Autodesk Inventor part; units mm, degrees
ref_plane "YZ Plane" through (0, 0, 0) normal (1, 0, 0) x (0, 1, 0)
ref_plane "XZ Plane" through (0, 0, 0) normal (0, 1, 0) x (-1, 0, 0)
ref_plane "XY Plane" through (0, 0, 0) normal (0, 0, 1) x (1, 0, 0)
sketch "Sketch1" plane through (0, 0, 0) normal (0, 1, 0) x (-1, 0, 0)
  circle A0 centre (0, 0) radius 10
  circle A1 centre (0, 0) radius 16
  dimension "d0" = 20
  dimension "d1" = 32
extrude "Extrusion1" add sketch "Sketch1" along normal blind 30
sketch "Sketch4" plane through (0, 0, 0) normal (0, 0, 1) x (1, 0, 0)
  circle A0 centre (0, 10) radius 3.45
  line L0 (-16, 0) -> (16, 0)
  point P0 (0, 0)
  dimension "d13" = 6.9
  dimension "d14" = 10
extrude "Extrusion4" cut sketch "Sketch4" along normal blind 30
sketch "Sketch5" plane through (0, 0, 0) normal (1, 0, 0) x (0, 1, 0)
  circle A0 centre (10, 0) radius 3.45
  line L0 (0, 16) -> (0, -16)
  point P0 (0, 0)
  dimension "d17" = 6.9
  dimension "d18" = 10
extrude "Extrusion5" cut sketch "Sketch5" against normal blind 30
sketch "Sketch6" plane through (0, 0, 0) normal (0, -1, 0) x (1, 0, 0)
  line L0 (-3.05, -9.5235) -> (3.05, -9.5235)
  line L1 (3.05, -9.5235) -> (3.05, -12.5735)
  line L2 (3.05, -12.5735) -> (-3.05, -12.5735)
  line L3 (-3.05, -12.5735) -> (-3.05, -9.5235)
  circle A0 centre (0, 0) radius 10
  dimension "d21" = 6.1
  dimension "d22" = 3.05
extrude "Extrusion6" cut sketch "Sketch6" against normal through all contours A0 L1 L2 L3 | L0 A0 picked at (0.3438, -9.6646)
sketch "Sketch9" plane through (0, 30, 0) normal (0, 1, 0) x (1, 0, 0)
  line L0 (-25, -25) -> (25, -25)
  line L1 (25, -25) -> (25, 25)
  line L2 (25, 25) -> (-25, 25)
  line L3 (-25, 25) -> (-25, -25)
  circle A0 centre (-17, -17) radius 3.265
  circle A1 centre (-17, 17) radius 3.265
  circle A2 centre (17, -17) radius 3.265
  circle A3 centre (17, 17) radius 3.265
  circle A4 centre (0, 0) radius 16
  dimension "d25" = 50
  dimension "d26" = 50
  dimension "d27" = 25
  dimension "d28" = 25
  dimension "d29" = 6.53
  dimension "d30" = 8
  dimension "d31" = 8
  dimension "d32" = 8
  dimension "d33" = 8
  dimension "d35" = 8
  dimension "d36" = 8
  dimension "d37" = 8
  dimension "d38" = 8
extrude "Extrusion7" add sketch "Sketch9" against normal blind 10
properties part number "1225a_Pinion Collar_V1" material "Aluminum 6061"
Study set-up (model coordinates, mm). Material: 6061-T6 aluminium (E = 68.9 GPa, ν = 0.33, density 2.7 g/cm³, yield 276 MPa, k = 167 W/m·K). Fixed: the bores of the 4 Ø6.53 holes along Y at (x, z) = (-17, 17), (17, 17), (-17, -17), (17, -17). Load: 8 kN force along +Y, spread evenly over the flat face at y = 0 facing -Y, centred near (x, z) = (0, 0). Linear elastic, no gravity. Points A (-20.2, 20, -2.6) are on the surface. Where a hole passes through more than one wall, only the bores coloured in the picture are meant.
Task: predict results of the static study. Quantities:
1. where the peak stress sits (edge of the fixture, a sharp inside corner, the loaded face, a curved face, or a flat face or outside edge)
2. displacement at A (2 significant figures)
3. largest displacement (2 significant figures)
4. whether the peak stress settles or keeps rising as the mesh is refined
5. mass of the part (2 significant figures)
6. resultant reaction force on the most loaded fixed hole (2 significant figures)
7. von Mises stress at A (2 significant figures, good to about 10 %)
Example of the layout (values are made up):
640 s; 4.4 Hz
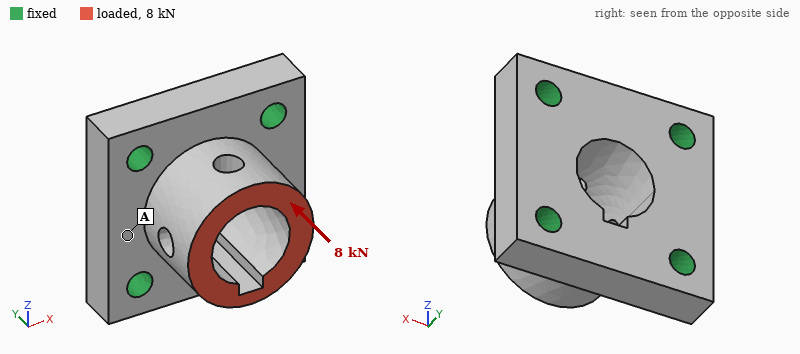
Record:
edge of the fixture; 3.9 µm; 14 µm; keeps rising; 79 g; 2.1 kN; 10 MPa
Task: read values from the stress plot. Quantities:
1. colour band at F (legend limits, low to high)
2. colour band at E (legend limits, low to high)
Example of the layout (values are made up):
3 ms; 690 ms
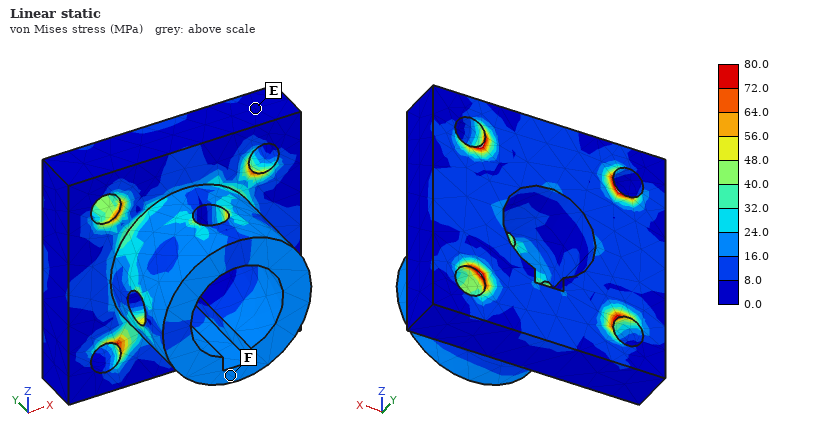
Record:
16.0 to 24.0 MPa; 0.0 to 8.0 MPa
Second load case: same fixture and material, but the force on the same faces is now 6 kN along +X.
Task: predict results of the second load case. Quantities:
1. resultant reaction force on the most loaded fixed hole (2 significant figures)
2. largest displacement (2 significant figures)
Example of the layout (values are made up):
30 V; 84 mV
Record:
2.9 kN; 60 µm
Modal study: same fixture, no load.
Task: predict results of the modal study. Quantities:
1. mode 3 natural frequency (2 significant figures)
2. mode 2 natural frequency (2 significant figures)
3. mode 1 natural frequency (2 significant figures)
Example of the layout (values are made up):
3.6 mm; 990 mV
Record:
23 kHz; 18 kHz; 18 kHz
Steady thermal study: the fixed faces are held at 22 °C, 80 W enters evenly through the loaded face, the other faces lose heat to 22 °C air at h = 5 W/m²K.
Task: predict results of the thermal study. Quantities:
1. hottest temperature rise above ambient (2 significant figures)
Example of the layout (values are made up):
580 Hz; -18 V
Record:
31 K
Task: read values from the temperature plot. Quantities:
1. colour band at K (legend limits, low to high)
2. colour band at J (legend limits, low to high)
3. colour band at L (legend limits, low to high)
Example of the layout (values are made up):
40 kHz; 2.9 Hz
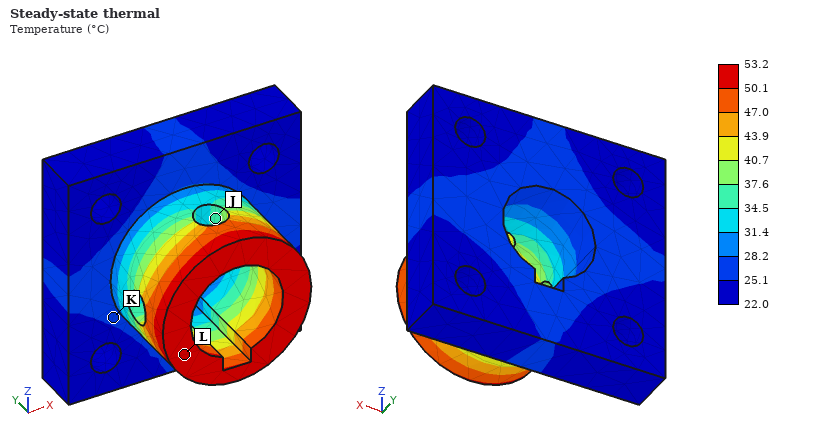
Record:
25.1 to 28.2 °C; 34.5 to 37.6 °C; 50.1 to 53.2 °C
